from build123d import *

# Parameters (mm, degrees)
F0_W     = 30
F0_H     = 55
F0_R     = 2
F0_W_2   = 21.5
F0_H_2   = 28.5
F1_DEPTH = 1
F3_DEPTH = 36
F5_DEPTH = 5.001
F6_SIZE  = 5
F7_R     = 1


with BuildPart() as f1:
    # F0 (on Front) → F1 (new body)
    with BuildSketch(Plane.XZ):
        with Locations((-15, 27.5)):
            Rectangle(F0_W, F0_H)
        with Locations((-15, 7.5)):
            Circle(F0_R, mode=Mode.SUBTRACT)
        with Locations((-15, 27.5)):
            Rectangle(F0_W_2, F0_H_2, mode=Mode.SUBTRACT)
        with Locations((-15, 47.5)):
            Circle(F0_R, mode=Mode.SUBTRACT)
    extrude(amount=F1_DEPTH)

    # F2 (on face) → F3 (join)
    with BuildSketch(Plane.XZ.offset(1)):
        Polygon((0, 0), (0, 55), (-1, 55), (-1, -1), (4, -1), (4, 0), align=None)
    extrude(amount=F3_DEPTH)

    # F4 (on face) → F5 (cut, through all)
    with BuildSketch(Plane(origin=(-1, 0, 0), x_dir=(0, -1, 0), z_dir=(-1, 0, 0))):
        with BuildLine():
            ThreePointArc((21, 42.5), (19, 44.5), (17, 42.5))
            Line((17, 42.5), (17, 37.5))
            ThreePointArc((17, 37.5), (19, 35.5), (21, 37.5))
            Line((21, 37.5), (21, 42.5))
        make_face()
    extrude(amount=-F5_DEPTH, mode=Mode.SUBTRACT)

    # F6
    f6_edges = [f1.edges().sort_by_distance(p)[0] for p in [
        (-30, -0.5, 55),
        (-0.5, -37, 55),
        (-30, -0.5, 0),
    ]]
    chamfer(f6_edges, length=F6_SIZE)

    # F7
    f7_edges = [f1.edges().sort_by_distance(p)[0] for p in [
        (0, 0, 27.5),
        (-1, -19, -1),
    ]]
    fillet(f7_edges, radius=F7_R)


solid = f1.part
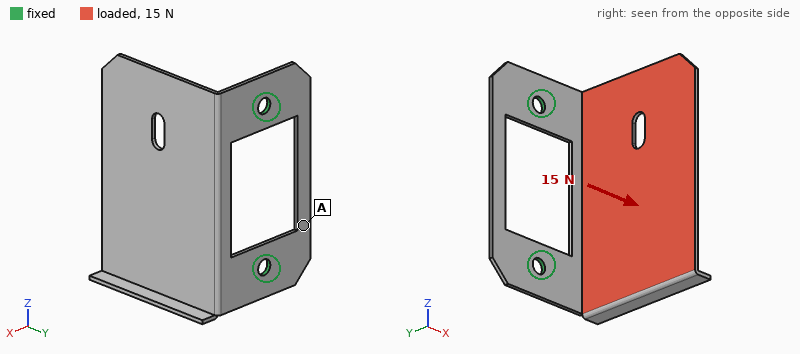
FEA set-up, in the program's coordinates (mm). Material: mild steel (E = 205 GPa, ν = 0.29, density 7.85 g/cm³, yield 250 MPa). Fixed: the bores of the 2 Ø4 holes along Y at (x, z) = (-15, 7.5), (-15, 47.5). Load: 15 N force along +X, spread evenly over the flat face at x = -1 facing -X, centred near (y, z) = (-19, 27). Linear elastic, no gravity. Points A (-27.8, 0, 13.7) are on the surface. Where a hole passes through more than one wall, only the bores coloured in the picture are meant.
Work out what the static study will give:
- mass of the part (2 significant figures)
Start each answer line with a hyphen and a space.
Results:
- 24 g
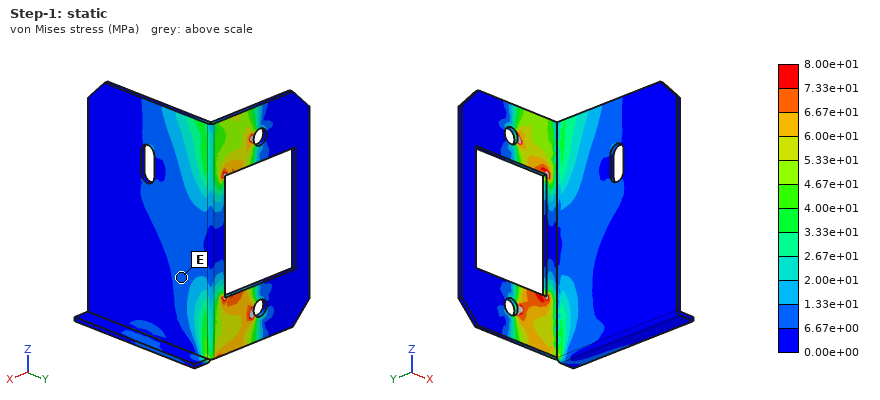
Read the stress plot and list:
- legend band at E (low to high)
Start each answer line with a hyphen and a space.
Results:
- 6.67e+00 to 1.33e+01 MPa
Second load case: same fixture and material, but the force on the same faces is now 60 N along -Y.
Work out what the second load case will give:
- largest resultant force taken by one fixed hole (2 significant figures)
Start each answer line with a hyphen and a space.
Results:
- 31 N
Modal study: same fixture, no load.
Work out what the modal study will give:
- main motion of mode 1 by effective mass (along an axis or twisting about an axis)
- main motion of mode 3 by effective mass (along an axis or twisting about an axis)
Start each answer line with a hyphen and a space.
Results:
- along X
- along Z
